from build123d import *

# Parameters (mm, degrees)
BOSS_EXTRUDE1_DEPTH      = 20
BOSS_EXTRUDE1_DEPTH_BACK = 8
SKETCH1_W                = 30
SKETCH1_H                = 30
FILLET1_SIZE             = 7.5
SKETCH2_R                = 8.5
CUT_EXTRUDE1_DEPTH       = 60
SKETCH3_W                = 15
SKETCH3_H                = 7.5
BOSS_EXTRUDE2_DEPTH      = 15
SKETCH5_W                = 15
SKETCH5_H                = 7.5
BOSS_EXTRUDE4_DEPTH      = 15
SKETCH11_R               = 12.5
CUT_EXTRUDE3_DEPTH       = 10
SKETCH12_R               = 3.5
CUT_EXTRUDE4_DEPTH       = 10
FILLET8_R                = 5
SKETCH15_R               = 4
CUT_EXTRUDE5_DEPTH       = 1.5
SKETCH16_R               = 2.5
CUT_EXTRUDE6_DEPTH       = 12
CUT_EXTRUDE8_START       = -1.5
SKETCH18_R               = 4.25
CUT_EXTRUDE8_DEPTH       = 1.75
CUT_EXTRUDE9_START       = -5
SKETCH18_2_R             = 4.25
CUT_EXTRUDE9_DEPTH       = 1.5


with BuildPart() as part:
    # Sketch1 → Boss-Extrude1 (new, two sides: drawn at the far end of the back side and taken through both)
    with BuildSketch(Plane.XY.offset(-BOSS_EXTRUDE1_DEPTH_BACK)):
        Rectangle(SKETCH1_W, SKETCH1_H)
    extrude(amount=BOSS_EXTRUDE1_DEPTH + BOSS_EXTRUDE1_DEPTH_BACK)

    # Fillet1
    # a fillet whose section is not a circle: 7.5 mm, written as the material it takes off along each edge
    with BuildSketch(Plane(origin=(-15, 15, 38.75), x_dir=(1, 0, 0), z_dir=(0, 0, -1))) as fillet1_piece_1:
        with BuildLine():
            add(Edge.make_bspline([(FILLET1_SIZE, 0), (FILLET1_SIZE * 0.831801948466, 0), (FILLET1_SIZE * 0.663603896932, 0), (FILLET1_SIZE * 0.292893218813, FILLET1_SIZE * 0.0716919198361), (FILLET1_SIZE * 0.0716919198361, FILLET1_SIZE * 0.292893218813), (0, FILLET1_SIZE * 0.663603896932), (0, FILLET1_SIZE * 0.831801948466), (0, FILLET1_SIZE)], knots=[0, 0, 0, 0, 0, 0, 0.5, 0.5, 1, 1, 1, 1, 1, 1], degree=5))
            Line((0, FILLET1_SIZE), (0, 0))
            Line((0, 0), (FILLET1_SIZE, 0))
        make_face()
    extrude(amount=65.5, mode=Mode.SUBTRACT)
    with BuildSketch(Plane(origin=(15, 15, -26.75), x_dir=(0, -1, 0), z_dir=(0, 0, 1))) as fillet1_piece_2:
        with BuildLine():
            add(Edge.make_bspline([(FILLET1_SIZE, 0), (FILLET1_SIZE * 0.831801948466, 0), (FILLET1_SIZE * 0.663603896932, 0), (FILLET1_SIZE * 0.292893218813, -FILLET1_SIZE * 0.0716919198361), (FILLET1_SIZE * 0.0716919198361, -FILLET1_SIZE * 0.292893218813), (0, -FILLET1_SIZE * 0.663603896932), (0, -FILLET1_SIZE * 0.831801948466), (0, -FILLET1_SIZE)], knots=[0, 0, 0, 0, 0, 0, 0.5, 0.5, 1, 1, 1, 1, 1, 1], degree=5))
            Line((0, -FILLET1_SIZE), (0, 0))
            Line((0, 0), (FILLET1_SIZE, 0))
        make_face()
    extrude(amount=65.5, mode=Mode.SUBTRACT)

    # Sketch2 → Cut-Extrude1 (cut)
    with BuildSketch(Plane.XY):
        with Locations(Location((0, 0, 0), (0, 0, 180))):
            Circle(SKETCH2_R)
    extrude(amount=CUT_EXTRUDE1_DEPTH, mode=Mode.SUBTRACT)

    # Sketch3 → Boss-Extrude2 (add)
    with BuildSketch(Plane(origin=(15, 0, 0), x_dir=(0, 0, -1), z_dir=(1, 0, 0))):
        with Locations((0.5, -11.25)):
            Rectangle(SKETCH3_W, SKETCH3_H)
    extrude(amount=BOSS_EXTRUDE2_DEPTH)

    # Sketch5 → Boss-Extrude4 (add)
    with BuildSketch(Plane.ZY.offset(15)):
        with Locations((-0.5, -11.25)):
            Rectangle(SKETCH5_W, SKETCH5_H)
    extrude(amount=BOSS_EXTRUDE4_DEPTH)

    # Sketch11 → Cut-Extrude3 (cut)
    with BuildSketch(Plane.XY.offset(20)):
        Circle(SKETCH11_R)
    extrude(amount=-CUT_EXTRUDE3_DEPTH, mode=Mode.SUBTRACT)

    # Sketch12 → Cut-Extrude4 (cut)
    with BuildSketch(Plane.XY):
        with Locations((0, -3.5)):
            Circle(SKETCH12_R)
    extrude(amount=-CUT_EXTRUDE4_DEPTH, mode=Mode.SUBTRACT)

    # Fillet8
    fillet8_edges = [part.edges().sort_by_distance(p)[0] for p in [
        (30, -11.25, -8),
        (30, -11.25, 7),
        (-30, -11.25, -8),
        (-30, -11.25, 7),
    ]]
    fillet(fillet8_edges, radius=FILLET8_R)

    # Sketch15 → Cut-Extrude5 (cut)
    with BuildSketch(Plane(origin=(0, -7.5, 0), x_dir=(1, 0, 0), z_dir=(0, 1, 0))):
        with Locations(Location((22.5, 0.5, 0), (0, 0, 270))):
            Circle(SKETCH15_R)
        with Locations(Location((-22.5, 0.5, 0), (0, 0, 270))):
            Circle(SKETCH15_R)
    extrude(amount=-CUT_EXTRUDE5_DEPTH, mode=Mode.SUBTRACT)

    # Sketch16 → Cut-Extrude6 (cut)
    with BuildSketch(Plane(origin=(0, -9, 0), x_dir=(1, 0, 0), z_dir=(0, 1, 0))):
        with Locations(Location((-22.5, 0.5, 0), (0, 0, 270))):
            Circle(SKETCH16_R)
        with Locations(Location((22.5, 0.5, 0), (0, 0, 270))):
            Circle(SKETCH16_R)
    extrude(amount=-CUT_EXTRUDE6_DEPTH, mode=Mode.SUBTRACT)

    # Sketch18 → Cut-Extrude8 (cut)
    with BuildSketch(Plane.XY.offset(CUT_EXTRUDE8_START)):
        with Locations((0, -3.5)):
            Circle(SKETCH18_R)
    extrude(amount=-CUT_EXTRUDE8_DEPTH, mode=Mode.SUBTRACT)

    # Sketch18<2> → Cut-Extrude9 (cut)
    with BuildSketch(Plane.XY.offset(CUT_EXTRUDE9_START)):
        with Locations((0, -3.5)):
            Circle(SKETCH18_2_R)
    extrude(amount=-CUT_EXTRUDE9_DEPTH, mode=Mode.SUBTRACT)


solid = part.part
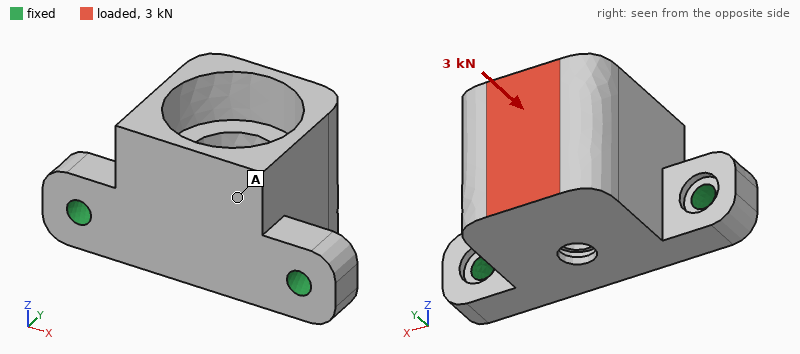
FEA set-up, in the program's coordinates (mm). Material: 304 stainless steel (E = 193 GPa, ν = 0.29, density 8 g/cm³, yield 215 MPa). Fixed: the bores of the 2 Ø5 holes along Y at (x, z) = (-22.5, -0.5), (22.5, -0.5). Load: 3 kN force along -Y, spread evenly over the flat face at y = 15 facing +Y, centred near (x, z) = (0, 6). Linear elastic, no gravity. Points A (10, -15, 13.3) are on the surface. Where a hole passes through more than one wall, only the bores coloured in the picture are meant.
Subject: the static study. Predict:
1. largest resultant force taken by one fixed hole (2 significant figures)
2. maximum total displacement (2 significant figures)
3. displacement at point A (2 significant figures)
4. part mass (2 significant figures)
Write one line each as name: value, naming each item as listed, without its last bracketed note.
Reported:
largest resultant force taken by one fixed hole: 1.6 kN
maximum total displacement: 40 µm
displacement at point A: 16 µm
part mass: 160 g
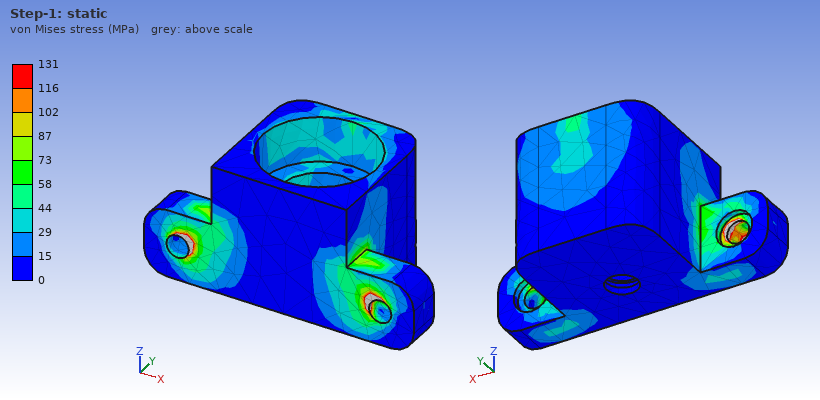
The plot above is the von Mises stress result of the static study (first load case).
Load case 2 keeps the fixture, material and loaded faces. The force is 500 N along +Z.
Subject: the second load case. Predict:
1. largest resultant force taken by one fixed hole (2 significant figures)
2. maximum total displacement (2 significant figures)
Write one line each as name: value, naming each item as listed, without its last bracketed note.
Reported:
largest resultant force taken by one fixed hole: 260 N
maximum total displacement: 22 µm
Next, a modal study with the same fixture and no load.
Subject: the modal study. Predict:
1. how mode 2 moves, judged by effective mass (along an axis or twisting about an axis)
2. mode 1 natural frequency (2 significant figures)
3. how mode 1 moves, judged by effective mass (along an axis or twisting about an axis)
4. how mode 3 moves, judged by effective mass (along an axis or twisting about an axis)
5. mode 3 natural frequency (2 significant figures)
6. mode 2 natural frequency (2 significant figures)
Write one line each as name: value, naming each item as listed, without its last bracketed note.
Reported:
how mode 2 moves, judged by effective mass: along X
mode 1 natural frequency: 3600 Hz
how mode 1 moves, judged by effective mass: along Z
how mode 3 moves, judged by effective mass: along Y
mode 3 natural frequency: 11 kHz
mode 2 natural frequency: 10 kHz
